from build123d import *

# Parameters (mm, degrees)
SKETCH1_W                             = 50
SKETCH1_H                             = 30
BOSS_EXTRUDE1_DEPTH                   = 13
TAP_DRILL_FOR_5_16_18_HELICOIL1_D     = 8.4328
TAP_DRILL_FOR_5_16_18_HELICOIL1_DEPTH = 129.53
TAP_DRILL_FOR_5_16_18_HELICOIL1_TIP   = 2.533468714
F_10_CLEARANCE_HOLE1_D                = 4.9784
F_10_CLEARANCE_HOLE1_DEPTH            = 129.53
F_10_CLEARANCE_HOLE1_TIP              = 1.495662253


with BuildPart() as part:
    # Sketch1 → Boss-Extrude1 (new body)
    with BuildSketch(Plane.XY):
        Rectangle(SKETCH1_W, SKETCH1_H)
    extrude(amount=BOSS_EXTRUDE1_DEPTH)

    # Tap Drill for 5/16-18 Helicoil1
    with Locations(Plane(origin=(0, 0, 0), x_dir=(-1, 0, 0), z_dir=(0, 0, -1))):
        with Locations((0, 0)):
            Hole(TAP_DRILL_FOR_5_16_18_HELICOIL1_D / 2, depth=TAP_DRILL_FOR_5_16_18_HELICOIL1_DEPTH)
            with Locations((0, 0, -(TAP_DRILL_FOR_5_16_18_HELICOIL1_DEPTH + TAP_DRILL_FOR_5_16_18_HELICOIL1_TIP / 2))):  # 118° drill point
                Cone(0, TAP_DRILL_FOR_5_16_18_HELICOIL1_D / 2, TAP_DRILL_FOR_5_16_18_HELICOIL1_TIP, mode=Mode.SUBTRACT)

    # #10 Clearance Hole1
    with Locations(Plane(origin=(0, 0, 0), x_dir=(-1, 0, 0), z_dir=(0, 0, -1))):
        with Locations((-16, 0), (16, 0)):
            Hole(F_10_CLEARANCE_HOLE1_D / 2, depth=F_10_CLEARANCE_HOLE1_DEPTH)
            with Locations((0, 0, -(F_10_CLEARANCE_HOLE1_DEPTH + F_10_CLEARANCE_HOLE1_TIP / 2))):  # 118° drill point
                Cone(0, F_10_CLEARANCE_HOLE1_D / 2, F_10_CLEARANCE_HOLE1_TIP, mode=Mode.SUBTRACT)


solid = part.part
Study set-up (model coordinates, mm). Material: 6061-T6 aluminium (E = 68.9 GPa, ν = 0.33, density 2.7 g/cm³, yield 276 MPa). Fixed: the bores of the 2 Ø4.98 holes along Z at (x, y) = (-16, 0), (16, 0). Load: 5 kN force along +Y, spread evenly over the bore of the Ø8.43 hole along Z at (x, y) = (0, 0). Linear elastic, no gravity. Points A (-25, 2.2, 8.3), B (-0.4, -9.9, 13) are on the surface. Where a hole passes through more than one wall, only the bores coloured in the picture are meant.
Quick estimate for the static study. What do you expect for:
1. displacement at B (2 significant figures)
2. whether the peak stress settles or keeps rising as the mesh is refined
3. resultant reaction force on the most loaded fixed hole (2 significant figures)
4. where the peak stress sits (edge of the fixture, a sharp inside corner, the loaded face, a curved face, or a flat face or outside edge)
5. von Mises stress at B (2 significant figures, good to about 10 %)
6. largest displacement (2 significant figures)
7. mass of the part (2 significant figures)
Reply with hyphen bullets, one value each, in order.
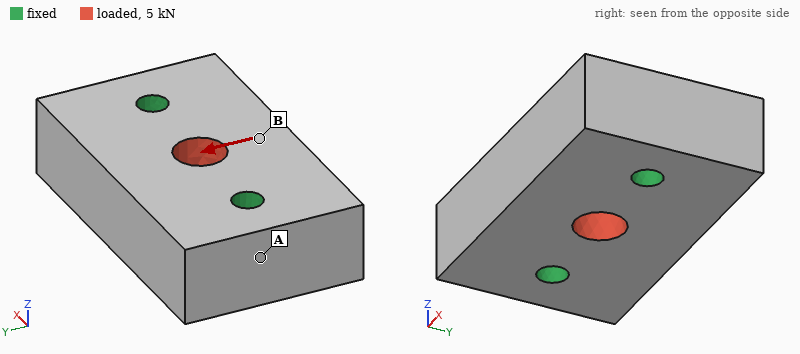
- 4.9 µm
- keeps rising
- 2.5 kN
- edge of the fixture
- 12 MPa
- 5.8 µm
- 49 g
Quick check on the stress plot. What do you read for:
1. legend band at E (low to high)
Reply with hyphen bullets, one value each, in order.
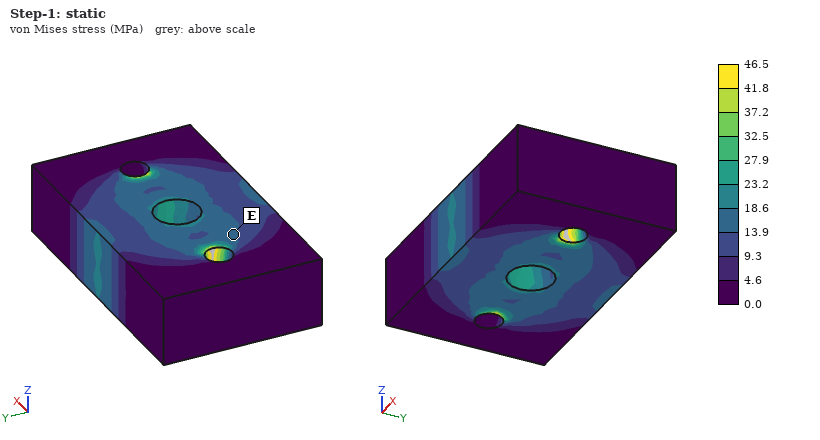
- 13.9 to 18.6 MPa
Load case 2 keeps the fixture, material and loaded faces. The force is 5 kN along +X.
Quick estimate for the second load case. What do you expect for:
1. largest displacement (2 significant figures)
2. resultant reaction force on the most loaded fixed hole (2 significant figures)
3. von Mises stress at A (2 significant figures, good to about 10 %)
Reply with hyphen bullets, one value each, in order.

- 3.0 µm
- 2.5 kN
- 5.5 MPa
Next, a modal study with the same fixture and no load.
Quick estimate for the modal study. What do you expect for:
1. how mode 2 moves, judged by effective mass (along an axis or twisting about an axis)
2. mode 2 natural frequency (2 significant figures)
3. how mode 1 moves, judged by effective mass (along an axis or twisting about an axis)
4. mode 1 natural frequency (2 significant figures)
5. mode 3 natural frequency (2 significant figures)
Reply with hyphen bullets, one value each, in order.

- along Z
- 28 kHz
- twisting about X
- 24 kHz
- 34 kHz
